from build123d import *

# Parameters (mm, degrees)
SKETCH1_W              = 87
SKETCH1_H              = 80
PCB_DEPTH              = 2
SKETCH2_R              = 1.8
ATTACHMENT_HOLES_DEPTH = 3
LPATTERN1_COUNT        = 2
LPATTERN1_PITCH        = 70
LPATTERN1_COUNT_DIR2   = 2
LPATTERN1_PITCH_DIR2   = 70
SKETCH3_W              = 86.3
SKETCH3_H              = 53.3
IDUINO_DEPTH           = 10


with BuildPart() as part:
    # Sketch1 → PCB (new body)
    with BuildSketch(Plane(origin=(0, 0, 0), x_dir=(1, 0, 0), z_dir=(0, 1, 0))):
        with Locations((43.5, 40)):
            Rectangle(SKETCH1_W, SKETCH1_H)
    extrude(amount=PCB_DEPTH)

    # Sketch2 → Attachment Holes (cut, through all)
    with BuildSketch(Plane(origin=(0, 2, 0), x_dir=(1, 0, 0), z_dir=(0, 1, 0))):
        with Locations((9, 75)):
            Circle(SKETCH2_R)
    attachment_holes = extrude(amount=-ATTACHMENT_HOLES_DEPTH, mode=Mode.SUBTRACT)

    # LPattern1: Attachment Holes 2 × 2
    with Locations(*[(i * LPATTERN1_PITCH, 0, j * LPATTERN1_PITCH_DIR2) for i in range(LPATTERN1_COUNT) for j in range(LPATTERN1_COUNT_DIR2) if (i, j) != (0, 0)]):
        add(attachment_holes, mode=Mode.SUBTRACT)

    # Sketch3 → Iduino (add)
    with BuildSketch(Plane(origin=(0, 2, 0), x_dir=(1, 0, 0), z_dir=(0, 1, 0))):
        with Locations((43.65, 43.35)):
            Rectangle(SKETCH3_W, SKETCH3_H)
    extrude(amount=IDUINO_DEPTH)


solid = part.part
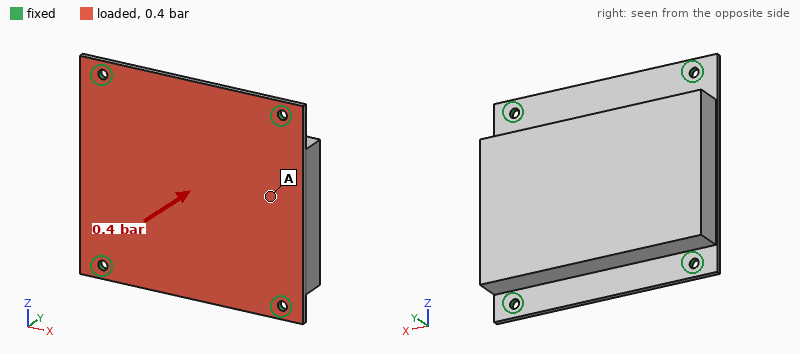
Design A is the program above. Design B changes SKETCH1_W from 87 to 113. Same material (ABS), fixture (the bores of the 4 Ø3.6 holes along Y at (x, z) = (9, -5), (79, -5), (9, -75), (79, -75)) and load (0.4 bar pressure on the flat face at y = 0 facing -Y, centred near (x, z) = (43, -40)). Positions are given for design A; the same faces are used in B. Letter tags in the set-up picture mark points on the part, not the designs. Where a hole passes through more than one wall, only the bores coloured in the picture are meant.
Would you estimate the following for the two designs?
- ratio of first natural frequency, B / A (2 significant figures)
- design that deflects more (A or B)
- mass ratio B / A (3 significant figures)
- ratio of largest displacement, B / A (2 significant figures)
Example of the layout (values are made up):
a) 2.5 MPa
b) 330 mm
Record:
a) 1.0
b) B
c) 1.07
d) 1.1
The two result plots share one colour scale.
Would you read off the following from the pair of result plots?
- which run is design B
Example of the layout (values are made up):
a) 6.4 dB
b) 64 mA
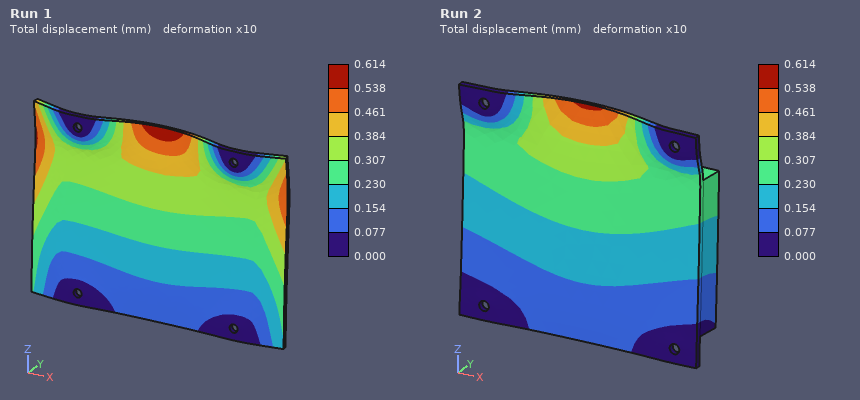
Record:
a) Run 1
